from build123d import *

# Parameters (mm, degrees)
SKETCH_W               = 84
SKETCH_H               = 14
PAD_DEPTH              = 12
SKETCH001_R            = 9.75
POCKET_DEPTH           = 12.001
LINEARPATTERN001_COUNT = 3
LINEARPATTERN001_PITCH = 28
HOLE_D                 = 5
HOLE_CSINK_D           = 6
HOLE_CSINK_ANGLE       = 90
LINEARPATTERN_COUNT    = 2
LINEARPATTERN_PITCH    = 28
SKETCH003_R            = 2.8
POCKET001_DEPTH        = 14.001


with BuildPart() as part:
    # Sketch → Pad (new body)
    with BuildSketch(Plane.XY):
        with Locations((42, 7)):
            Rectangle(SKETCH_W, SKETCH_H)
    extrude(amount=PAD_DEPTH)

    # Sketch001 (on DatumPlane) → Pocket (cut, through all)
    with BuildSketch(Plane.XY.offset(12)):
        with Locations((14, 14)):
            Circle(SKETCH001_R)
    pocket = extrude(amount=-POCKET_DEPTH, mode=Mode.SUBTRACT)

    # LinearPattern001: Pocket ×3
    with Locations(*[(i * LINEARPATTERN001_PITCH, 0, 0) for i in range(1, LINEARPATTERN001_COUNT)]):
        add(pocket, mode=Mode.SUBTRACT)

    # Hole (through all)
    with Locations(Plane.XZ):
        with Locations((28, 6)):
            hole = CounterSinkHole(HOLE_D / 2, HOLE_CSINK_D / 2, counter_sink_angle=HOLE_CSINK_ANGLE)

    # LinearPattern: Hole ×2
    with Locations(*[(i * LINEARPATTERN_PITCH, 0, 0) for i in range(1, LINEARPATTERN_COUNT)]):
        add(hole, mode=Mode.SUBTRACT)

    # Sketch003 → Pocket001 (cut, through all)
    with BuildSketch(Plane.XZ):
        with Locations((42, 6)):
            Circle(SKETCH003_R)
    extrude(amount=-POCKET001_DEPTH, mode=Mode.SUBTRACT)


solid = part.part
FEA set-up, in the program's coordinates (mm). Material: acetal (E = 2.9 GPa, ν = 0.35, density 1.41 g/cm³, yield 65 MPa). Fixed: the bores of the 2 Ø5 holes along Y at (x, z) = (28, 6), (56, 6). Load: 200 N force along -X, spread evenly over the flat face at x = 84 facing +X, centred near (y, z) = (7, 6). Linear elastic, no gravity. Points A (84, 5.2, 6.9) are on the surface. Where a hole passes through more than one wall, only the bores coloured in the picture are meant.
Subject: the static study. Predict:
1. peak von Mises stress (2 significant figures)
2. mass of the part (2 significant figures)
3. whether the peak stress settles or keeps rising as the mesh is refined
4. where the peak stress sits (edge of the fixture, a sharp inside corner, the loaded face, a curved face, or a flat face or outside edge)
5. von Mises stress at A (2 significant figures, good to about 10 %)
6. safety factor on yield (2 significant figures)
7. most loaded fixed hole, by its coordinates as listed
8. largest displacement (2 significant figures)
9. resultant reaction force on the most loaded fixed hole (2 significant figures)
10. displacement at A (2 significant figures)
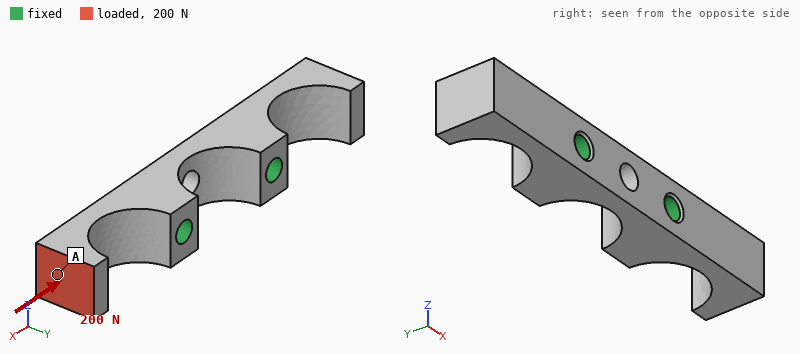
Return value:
32 MPa
11 g
settles
a curved face
3.4 MPa
2.0
(56, 6)
0.83 mm
200 N
0.64 mm
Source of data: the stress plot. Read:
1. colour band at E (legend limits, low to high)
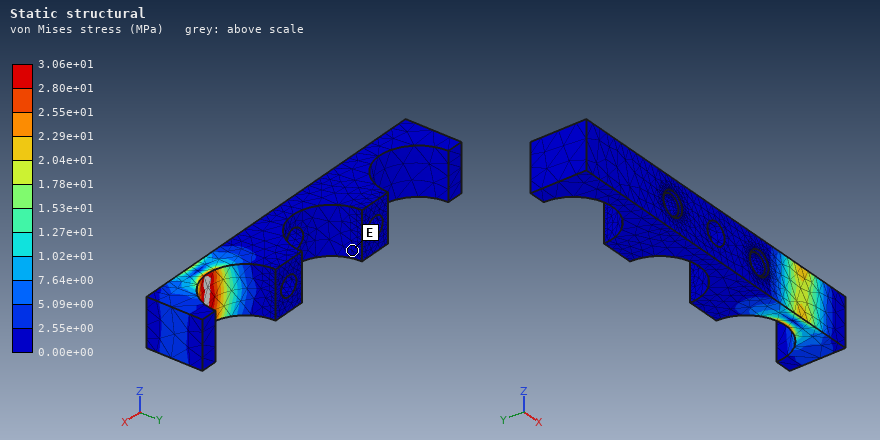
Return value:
0.00e+00 to 2.55e+00 MPa
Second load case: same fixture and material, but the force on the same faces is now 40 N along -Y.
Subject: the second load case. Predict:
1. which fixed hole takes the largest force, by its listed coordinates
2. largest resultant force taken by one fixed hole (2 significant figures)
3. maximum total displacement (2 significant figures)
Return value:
(56, 6)
41 N
0.56 mm
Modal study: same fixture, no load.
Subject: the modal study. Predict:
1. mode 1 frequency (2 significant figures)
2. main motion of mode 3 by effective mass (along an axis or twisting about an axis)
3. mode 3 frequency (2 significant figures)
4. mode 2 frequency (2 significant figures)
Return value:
1400 Hz
along Z
2100 Hz
1400 Hz
